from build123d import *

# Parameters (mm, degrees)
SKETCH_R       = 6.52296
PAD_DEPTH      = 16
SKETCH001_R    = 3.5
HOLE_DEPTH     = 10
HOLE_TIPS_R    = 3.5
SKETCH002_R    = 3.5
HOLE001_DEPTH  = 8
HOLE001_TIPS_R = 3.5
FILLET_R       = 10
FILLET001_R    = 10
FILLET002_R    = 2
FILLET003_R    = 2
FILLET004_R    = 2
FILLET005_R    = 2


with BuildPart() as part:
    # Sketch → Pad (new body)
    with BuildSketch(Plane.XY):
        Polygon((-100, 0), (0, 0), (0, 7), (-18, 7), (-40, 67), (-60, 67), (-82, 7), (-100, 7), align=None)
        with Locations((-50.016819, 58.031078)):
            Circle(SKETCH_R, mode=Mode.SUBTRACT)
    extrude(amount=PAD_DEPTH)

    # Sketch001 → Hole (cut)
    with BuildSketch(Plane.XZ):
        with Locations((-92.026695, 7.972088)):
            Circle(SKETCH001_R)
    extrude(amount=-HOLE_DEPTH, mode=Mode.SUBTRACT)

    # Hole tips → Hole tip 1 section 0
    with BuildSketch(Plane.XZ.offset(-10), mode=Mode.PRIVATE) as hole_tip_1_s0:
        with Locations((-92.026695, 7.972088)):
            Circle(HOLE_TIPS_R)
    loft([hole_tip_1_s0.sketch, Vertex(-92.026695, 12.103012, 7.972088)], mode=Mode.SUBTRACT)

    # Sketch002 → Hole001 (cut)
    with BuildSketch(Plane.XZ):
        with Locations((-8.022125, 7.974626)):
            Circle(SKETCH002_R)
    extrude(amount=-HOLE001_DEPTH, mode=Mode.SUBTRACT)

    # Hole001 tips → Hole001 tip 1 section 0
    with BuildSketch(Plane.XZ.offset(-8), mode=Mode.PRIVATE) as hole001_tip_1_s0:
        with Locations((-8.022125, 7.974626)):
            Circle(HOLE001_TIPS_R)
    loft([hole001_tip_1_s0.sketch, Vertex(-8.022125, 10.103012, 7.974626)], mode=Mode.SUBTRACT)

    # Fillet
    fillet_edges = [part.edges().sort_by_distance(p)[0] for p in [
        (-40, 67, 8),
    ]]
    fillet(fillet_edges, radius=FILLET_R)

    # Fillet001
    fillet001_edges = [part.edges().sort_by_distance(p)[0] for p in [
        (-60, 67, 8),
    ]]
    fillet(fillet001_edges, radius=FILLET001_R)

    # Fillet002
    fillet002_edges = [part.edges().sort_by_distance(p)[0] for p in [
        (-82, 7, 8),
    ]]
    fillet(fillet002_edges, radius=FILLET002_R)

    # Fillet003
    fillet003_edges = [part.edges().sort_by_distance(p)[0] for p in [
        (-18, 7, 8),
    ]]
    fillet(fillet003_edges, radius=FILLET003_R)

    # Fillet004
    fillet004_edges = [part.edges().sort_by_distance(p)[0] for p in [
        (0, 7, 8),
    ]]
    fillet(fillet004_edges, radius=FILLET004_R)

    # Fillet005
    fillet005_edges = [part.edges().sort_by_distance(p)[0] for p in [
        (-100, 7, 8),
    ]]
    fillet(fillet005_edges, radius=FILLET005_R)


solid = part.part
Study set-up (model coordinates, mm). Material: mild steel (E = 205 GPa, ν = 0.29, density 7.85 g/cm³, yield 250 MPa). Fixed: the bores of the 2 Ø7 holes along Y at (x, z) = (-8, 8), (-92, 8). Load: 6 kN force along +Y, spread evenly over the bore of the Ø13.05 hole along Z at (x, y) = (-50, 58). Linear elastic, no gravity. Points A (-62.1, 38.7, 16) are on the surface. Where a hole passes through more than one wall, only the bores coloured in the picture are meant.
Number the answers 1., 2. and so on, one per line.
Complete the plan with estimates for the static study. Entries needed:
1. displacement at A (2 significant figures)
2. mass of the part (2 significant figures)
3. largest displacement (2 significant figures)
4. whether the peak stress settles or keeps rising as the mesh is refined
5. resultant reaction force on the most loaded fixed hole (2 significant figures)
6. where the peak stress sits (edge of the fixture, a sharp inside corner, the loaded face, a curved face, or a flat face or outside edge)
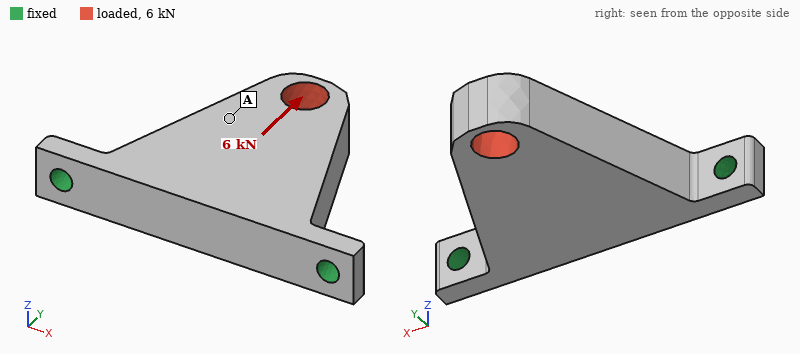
1. 12 µm
2. 380 g
3. 16 µm
4. keeps rising
5. 3.6 kN
6. edge of the fixture
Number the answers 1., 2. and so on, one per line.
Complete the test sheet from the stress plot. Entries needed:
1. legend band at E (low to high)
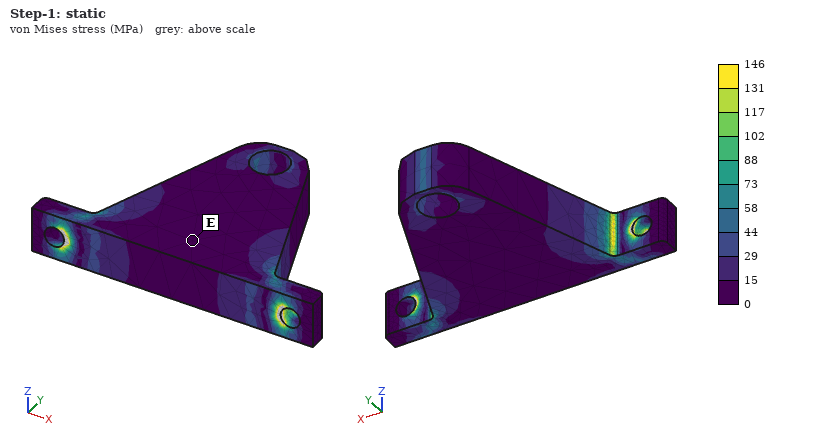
1. 0 to 15 MPa
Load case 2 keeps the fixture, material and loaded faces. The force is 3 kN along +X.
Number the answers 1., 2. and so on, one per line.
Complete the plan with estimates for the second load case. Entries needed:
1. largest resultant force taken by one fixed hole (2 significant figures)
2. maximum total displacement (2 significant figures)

1. 2.8 kN
2. 23 µm
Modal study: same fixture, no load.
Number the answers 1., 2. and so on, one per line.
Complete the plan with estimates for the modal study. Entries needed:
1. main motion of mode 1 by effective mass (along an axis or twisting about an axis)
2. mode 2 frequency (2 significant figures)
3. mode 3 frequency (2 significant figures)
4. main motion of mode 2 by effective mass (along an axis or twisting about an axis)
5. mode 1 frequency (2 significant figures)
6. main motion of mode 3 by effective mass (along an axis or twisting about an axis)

1. along Z
2. 6200 Hz
3. 6600 Hz
4. along Y
5. 1400 Hz
6. along X
